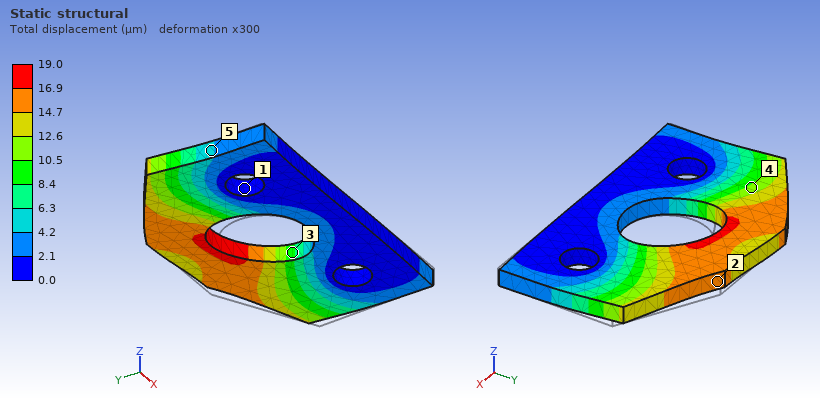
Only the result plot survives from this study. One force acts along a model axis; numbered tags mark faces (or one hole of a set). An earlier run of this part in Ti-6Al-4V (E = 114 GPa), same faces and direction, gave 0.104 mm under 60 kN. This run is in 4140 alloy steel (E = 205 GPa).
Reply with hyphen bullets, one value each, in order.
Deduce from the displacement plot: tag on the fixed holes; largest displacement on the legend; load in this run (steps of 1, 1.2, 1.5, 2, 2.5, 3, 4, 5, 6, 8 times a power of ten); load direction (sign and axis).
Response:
- 1
- 19.0 µm
- 20 kN
- -X
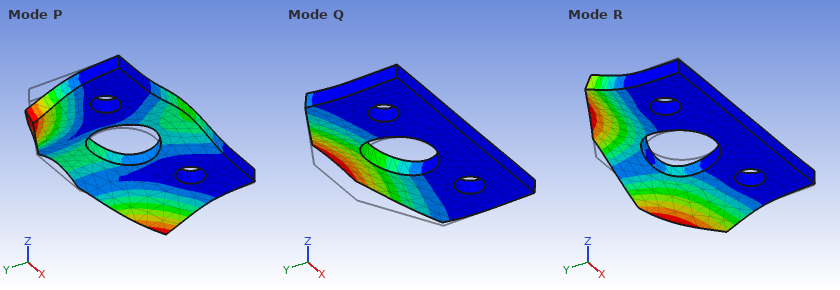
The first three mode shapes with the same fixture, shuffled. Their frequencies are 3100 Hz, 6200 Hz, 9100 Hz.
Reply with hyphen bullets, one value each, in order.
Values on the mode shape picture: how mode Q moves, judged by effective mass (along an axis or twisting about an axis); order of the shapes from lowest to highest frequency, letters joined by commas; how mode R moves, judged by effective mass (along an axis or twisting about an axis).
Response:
- along Z
- Q, R, P
- twisting about Y
